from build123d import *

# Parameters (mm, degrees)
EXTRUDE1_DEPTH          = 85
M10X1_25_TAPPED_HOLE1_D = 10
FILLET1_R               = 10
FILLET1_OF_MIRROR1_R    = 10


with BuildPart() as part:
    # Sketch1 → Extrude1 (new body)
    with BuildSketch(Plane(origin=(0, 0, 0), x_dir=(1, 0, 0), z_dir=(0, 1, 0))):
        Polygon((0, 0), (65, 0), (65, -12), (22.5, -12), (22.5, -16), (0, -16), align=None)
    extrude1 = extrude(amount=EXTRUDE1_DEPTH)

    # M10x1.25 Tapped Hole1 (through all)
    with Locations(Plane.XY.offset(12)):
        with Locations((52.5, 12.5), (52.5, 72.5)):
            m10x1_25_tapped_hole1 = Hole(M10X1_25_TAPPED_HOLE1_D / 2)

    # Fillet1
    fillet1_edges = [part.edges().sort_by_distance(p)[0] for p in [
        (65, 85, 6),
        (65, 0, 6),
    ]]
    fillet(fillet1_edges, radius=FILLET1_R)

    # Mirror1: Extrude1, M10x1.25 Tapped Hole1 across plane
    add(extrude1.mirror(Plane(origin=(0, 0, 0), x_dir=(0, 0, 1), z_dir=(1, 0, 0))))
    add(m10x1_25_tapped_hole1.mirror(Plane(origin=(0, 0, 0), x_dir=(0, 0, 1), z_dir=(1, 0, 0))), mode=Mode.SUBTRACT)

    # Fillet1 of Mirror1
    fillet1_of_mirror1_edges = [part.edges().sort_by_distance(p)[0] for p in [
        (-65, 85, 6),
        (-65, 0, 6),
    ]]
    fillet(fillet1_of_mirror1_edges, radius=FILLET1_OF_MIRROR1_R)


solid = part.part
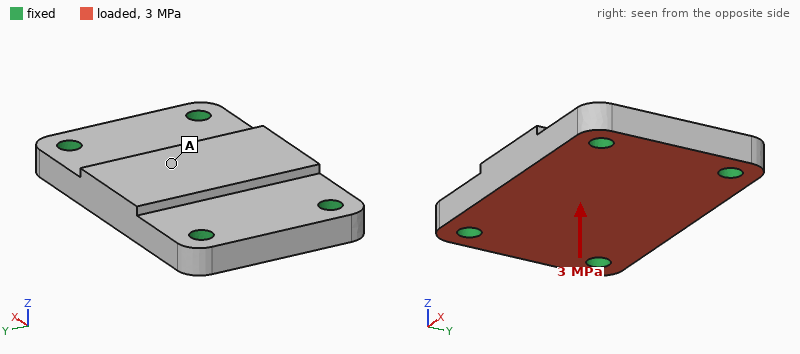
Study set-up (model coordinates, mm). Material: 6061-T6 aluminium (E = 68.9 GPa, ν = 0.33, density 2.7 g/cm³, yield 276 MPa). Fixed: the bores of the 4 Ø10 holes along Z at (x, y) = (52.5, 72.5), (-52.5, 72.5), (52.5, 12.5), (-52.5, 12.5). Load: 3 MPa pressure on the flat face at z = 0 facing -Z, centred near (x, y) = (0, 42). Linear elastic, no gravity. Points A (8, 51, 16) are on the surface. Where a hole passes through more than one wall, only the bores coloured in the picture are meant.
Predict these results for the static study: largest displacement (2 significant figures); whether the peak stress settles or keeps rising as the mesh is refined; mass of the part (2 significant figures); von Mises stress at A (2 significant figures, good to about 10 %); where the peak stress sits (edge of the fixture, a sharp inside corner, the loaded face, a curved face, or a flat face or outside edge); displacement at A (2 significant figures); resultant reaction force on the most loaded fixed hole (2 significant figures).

84 µm
keeps rising
390 g
33 MPa
edge of the fixture
81 µm
8.1 kN
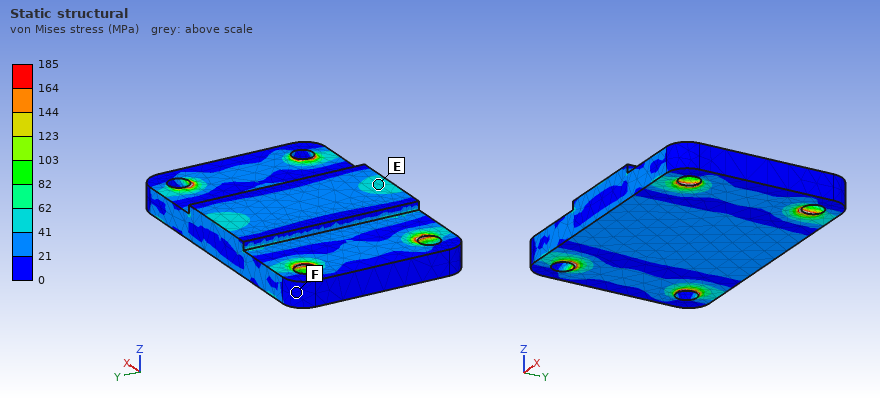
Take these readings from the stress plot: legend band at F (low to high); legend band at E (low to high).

0 to 21 MPa
41 to 62 MPa
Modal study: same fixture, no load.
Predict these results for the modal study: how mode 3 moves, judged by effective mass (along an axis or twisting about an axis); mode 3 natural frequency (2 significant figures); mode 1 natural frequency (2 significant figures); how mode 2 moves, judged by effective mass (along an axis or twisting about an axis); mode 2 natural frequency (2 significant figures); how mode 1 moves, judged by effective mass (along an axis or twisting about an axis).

along Y
12 kHz
5300 Hz
twisting about X
6800 Hz
along Z
